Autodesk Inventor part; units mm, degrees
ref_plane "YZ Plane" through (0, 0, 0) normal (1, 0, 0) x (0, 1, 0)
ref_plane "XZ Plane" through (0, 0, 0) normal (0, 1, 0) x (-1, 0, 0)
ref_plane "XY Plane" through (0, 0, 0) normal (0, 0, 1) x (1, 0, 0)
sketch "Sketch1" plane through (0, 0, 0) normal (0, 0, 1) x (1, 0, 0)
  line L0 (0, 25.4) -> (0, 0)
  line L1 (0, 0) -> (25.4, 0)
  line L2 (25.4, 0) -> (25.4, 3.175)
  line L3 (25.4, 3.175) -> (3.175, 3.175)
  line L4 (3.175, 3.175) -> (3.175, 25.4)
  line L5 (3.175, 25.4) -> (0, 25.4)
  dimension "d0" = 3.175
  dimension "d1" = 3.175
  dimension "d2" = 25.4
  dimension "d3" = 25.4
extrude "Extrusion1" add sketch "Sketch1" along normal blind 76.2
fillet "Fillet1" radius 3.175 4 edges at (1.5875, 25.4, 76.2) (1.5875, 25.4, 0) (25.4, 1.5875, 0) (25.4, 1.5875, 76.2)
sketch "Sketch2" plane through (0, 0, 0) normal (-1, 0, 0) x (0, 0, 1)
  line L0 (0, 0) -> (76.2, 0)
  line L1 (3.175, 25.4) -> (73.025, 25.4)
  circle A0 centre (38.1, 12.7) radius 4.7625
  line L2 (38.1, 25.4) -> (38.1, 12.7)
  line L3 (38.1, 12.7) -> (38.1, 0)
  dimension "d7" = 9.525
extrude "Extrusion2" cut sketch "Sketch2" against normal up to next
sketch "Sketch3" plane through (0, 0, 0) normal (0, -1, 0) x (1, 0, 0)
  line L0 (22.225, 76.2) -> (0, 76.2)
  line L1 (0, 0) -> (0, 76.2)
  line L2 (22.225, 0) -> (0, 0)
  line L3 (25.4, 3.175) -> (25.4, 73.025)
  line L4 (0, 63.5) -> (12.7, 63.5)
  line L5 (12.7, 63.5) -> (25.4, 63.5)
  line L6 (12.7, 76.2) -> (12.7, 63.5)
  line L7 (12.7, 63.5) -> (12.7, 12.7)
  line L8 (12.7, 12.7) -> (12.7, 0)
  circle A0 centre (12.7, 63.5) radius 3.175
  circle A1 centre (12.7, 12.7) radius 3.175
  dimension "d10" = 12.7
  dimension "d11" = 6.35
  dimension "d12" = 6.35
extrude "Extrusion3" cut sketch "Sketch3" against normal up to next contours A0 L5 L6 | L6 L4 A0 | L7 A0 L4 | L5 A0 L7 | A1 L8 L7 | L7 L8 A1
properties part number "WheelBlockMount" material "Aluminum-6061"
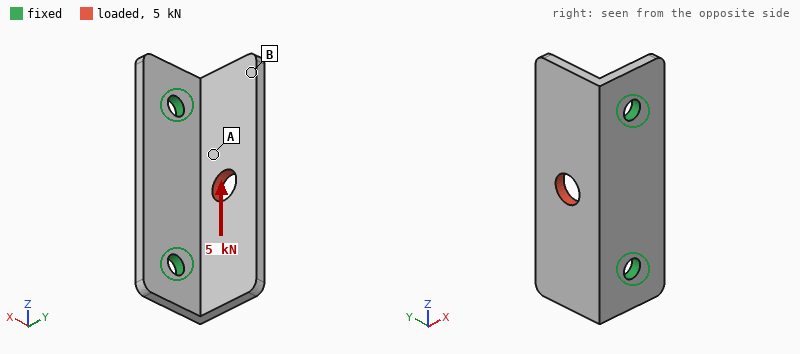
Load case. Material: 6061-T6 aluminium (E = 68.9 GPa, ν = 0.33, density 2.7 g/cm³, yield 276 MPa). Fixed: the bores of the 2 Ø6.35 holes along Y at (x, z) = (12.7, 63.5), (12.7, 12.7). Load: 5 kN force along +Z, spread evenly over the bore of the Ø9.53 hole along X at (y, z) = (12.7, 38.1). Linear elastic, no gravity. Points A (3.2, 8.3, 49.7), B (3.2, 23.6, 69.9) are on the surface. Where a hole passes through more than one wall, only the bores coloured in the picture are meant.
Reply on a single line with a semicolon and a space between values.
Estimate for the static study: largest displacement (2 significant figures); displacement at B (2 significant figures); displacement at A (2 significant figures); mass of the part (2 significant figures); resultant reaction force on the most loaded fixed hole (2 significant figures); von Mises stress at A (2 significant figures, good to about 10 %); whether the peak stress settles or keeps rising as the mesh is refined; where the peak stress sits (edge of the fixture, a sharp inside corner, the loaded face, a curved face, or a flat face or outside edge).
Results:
0.19 mm; 0.16 mm; 0.044 mm; 30 g; 2.9 kN; 78 MPa; keeps rising; edge of the fixture
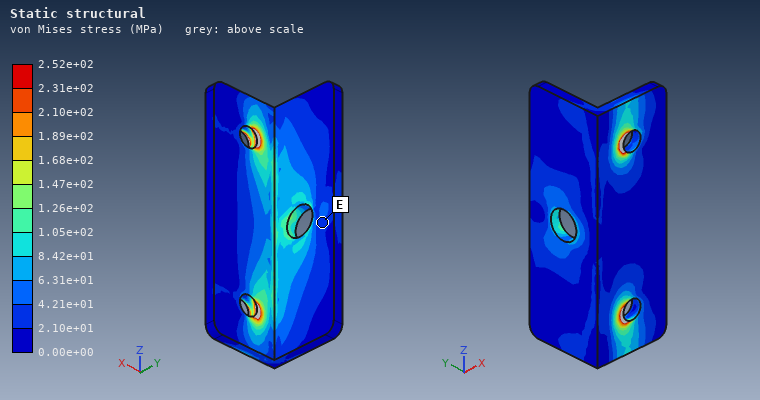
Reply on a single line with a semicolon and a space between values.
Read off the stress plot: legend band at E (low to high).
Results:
2.10e+01 to 4.21e+01 MPa
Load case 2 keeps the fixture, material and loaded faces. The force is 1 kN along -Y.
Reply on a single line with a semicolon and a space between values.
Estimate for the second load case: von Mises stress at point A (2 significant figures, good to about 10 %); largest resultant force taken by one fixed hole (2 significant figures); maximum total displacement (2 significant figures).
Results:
15 MPa; 540 N; 0.12 mm
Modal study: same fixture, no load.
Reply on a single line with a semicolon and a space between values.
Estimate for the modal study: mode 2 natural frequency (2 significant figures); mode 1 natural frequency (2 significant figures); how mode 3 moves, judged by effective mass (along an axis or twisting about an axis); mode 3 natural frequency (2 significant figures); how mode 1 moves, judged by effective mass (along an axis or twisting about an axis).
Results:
3900 Hz; 2700 Hz; along Y; 7000 Hz; along X
